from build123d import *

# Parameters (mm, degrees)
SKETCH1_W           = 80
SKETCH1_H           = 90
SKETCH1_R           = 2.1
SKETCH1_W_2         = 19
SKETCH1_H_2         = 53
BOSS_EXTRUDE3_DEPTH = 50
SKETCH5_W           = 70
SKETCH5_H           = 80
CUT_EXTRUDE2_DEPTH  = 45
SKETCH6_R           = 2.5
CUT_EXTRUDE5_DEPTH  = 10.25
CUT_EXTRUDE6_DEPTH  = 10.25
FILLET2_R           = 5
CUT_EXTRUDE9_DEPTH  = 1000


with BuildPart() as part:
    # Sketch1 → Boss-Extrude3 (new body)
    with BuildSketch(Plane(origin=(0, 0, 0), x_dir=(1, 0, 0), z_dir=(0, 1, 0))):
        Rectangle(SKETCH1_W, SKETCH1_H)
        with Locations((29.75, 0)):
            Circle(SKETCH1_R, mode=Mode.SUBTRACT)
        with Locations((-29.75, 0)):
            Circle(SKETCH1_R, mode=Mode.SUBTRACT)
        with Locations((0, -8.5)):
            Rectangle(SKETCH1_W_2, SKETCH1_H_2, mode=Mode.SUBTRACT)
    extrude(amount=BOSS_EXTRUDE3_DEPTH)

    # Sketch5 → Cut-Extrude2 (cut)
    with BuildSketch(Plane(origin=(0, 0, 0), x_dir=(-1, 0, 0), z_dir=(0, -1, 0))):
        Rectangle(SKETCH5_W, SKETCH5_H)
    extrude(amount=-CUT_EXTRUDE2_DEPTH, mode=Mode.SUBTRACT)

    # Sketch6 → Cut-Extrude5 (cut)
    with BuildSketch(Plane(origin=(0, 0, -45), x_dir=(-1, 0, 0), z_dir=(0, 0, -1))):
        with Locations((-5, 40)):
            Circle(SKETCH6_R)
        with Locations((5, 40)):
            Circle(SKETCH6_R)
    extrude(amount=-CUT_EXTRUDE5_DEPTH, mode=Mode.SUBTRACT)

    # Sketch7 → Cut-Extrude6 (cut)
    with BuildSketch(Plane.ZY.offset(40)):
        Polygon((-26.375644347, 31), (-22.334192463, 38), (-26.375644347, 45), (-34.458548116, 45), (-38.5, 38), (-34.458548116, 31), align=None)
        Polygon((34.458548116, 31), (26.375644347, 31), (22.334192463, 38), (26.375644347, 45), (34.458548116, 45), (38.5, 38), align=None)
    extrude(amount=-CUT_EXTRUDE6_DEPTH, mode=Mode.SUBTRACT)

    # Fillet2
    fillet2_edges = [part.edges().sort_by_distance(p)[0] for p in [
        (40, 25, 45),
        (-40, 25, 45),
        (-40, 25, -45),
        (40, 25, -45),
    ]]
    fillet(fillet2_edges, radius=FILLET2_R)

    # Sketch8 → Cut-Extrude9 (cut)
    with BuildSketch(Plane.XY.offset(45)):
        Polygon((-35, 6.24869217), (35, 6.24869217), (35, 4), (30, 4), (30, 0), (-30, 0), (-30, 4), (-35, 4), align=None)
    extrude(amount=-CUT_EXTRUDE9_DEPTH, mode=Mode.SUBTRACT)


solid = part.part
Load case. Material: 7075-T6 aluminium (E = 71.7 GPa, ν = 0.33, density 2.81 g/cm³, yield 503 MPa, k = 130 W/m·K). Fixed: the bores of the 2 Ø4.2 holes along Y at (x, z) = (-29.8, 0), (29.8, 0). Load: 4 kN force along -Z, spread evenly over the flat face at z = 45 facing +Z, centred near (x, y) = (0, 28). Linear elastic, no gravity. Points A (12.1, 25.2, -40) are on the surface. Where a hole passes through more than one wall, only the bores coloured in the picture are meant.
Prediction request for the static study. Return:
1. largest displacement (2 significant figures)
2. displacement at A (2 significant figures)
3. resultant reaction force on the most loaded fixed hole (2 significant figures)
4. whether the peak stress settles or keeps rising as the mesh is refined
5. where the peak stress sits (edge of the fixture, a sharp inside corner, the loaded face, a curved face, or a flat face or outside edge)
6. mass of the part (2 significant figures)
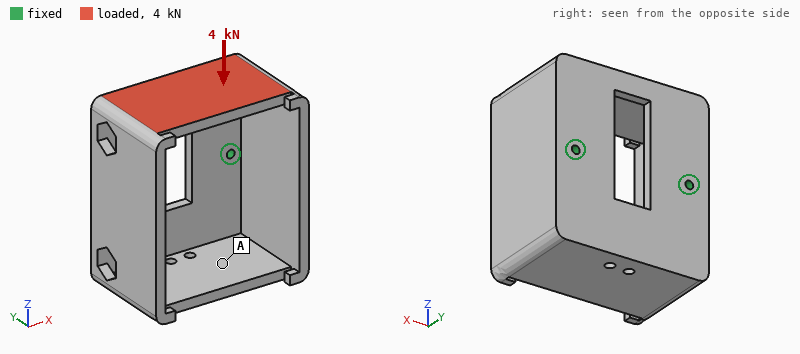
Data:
0.67 mm
0.37 mm
2.1 kN
keeps rising
edge of the fixture
270 g
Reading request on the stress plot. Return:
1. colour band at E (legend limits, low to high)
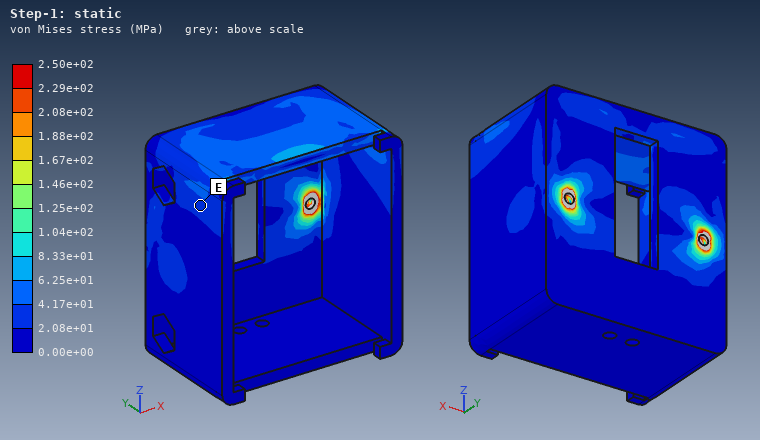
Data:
2.08e+01 to 4.17e+01 MPa
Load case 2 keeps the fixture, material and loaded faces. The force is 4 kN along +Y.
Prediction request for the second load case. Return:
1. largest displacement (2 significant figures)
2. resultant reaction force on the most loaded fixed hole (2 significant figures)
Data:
1.2 mm
2.1 kN
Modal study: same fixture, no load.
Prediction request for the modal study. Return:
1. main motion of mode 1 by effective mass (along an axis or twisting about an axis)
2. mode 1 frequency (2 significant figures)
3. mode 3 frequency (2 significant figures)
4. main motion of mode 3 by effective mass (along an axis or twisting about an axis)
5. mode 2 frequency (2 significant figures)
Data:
along Z
780 Hz
2600 Hz
along X
1500 Hz
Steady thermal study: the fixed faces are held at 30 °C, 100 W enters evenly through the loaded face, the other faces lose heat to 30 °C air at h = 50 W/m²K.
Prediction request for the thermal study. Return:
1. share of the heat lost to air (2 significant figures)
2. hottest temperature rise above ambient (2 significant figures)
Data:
42 %
68 K
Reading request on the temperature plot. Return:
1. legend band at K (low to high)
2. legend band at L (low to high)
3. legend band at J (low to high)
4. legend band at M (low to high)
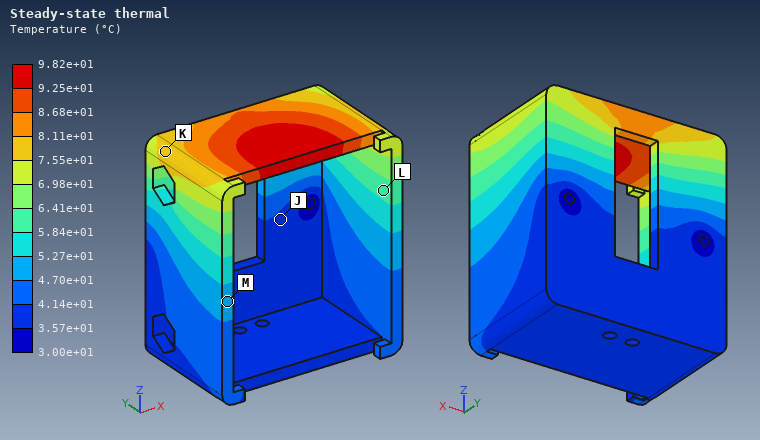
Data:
7.55e+01 to 8.11e+01 °C
5.84e+01 to 6.41e+01 °C
3.57e+01 to 4.14e+01 °C
4.70e+01 to 5.27e+01 °C
